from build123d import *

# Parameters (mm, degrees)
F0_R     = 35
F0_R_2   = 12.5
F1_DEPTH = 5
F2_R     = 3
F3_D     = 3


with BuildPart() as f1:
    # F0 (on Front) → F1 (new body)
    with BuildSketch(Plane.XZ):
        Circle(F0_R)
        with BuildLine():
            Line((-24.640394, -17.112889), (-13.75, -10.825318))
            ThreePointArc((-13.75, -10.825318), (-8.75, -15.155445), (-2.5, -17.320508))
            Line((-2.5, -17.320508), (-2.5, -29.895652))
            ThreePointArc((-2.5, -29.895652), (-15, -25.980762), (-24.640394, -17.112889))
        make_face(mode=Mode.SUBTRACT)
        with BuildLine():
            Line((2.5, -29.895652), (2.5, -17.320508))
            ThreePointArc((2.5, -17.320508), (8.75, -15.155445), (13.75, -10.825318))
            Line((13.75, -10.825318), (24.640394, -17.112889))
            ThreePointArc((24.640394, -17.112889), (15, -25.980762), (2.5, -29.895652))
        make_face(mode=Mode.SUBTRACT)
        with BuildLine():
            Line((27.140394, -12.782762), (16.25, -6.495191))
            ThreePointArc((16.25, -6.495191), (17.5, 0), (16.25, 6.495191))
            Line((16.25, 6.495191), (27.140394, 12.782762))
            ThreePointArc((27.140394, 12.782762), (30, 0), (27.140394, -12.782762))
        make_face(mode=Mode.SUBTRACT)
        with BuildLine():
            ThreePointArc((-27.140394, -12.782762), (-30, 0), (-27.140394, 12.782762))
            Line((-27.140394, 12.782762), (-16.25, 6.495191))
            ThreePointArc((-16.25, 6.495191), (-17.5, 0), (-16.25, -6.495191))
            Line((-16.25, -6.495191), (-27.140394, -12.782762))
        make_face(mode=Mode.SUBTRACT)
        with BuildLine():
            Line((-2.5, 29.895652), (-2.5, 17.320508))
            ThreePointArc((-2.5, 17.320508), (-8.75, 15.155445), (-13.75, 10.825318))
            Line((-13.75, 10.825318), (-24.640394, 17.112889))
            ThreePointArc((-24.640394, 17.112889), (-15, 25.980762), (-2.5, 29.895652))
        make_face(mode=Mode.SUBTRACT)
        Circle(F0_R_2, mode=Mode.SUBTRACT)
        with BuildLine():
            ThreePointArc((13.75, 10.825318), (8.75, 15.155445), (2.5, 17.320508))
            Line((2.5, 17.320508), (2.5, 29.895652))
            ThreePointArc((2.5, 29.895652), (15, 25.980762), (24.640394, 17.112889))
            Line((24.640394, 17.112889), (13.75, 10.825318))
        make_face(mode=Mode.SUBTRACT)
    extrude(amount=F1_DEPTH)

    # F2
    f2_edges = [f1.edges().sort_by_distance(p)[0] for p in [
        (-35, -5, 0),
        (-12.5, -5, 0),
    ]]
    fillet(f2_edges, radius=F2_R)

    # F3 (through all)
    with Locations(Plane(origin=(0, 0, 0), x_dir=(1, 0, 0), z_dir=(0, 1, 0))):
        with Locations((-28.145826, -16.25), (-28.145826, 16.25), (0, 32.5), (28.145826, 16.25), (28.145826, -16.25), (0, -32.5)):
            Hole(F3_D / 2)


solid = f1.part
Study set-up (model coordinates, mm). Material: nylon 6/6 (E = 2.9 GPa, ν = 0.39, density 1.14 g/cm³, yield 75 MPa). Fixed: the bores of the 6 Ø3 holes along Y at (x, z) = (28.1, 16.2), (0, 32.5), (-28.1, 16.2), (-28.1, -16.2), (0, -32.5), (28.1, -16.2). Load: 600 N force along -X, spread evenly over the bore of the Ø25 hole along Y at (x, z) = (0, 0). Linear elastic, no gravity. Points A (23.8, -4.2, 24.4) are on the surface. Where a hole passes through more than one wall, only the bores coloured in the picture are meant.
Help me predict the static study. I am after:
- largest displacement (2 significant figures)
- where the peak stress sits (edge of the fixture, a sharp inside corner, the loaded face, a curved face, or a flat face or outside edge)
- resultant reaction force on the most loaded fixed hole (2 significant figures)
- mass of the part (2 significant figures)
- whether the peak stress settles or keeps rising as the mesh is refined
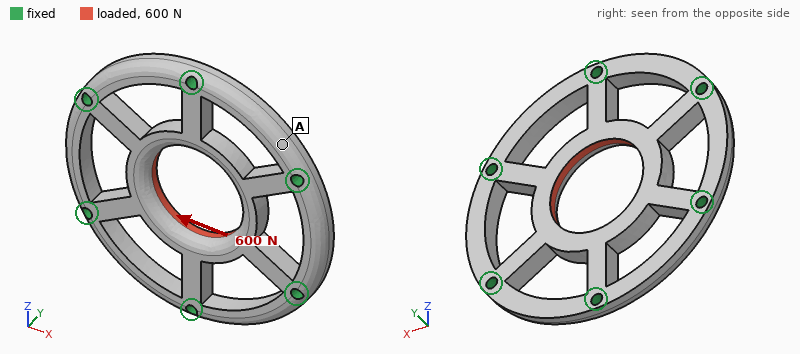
79 µm
edge of the fixture
160 N
9.8 g
keeps rising
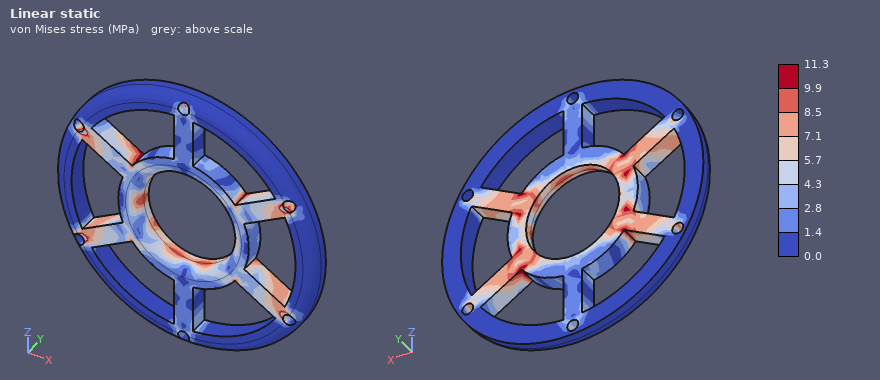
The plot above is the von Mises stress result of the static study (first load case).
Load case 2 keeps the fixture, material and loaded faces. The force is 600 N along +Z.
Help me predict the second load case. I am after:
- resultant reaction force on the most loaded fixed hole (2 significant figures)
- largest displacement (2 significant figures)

180 N
75 µm
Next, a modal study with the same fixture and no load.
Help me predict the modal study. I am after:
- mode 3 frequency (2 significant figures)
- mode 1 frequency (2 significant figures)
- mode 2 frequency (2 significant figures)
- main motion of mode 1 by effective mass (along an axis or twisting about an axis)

4200 Hz
2800 Hz
4200 Hz
along Y
